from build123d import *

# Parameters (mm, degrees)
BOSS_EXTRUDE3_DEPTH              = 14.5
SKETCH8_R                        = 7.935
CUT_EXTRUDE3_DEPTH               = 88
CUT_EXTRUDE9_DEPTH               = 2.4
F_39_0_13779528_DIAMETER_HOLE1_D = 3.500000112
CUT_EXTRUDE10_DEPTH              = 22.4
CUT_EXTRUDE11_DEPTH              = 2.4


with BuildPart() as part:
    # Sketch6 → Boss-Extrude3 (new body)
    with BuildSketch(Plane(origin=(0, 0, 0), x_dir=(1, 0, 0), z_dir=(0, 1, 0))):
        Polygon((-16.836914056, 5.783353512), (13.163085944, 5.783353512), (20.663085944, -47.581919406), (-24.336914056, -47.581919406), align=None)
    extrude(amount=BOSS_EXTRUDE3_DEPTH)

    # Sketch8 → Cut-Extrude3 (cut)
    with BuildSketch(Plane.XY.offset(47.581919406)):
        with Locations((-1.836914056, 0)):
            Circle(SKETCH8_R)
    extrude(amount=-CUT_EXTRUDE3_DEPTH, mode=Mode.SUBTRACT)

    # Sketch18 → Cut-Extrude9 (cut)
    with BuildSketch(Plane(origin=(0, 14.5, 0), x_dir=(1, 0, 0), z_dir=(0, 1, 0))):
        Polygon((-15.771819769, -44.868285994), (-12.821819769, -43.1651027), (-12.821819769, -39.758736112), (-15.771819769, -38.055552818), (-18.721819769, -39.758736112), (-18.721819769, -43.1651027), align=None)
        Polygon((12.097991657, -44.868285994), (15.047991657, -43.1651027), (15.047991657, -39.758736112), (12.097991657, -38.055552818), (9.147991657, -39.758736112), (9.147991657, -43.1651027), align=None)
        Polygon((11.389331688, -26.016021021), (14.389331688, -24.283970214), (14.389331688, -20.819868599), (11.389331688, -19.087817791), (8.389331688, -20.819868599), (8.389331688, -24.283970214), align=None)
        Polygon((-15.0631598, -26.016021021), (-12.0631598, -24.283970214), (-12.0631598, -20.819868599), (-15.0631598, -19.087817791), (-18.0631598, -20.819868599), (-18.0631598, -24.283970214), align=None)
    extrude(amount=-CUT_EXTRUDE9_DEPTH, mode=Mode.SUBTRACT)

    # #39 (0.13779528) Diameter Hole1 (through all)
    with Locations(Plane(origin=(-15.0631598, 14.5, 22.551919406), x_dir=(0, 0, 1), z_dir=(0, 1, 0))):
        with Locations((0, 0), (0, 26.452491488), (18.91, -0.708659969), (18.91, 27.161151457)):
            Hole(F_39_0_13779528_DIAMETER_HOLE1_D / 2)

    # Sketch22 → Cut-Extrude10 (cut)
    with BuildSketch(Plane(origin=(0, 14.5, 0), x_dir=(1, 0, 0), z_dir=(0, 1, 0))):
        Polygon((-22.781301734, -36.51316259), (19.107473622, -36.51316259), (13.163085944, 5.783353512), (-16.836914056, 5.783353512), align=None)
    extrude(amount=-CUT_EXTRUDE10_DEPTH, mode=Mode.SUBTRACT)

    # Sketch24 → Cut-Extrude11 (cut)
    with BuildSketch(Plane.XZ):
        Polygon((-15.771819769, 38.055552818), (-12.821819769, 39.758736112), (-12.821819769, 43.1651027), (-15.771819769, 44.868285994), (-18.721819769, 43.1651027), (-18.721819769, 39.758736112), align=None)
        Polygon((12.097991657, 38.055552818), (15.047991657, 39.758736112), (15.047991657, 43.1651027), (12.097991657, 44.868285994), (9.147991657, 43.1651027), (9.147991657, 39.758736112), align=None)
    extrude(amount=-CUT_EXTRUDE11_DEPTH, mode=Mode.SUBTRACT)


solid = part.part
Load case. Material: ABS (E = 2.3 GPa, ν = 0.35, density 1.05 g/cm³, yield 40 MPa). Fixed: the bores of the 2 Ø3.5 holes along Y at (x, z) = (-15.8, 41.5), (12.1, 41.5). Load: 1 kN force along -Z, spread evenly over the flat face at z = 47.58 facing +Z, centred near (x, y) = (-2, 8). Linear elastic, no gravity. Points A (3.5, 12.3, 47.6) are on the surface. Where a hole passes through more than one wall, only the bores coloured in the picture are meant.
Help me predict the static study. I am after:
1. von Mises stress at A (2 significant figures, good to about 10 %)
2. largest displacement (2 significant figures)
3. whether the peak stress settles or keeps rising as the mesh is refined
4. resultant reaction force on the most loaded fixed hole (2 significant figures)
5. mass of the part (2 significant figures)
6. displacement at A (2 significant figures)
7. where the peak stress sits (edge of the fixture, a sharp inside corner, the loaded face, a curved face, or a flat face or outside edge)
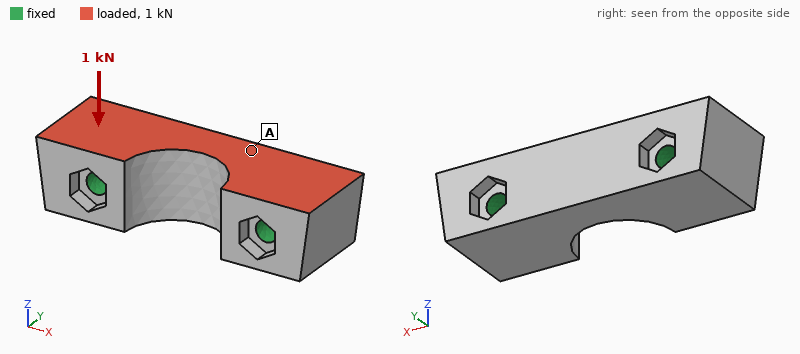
2.2 MPa
43 µm
keeps rising
500 N
5.7 g
34 µm
edge of the fixture
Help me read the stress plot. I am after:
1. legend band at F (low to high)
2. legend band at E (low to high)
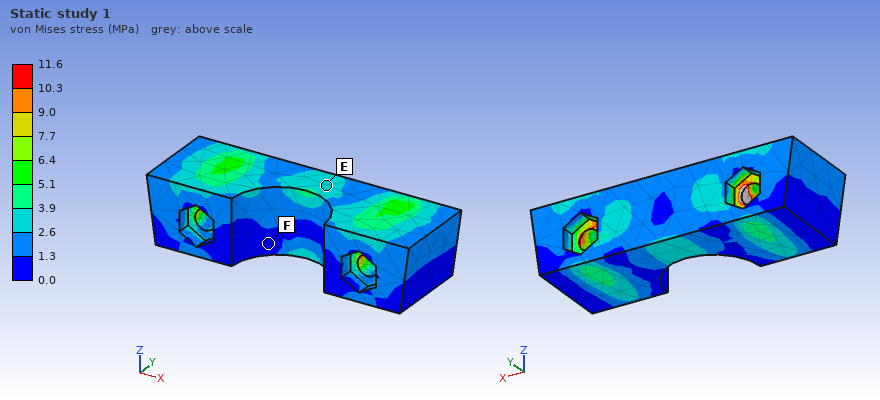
0.0 to 1.3 MPa
2.6 to 3.9 MPa
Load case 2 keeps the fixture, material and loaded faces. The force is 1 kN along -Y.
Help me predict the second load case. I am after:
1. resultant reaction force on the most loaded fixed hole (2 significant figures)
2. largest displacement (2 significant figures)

500 N
96 µm
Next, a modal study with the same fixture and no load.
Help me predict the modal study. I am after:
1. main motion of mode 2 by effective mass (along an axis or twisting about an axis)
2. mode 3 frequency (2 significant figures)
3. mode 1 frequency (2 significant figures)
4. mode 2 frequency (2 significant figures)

along Y
15 kHz
9900 Hz
13 kHz
